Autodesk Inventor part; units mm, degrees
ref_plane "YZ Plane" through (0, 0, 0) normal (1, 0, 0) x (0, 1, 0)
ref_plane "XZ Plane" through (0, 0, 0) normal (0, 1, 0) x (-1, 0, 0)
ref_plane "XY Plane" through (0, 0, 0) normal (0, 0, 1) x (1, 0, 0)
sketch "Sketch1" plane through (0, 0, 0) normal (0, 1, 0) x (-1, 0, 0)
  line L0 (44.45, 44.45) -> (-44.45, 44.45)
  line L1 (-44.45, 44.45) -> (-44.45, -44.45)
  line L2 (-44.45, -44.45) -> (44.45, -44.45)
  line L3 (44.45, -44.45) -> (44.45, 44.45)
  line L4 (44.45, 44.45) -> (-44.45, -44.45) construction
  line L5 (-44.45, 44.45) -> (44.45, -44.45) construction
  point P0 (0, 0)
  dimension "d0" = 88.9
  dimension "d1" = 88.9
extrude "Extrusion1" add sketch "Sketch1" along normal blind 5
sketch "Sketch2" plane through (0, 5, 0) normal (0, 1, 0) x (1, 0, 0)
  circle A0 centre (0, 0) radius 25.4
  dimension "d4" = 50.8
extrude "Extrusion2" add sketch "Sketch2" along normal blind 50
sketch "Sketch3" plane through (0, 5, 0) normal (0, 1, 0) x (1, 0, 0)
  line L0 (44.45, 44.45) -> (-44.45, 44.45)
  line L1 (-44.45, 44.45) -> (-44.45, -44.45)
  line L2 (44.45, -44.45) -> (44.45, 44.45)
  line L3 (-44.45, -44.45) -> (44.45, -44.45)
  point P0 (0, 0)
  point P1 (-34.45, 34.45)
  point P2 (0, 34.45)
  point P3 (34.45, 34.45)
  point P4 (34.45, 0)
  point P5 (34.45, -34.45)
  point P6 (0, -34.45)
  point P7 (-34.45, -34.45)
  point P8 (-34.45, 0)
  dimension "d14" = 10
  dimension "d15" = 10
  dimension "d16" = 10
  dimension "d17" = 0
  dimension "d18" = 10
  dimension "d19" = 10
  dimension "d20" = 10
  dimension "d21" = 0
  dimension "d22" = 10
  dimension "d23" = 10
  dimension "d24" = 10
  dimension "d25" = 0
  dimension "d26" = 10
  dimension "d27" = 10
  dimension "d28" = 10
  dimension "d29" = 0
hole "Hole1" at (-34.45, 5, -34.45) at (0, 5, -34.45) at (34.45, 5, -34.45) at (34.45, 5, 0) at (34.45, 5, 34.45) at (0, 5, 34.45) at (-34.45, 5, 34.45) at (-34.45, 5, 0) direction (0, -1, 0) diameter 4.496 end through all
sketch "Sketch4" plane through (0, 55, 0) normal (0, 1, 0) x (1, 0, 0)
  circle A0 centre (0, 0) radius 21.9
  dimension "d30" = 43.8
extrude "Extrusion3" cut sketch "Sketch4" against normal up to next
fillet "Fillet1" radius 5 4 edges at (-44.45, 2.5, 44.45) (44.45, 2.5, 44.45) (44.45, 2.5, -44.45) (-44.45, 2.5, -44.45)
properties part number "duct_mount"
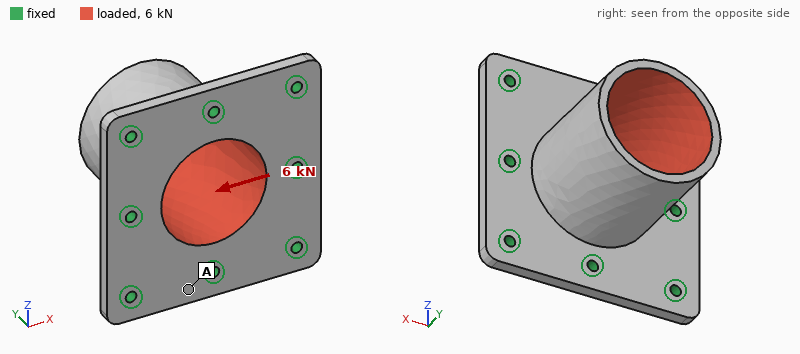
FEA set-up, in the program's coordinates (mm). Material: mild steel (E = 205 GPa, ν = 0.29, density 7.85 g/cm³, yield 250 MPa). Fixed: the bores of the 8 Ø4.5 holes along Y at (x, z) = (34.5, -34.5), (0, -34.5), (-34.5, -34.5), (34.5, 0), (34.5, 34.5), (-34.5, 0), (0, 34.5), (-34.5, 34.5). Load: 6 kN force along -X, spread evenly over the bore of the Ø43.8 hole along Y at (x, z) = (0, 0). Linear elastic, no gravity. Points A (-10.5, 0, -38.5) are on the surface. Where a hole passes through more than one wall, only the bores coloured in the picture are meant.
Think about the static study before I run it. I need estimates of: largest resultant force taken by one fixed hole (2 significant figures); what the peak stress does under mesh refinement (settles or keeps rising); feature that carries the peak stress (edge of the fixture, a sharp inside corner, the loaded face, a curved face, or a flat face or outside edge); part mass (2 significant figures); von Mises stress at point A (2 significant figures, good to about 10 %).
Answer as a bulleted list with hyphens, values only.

- 2.5 kN
- keeps rising
- edge of the fixture
- 450 g
- 11 MPa
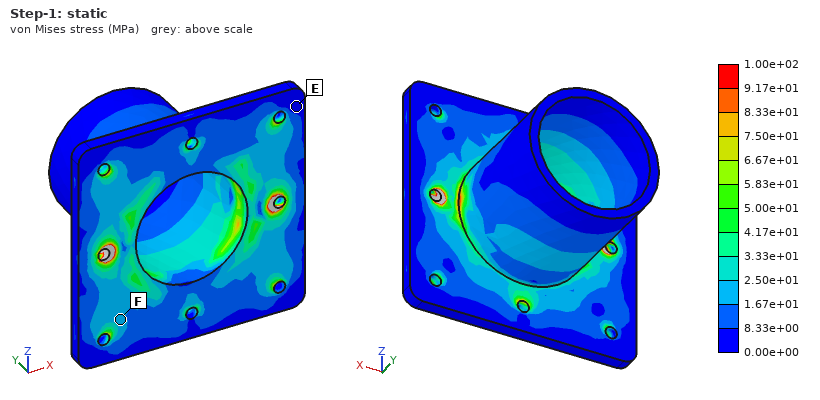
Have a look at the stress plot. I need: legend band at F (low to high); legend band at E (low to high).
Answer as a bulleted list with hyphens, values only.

- 1.67e+01 to 2.50e+01 MPa
- 0.00e+00 to 8.33e+00 MPa
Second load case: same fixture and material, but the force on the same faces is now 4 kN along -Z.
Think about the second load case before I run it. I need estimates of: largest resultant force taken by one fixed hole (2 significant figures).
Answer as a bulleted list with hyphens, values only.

- 1.7 kN
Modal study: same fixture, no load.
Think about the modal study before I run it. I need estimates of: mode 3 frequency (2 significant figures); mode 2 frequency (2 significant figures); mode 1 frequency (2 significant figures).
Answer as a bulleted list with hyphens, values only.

- 5100 Hz
- 4900 Hz
- 4900 Hz
